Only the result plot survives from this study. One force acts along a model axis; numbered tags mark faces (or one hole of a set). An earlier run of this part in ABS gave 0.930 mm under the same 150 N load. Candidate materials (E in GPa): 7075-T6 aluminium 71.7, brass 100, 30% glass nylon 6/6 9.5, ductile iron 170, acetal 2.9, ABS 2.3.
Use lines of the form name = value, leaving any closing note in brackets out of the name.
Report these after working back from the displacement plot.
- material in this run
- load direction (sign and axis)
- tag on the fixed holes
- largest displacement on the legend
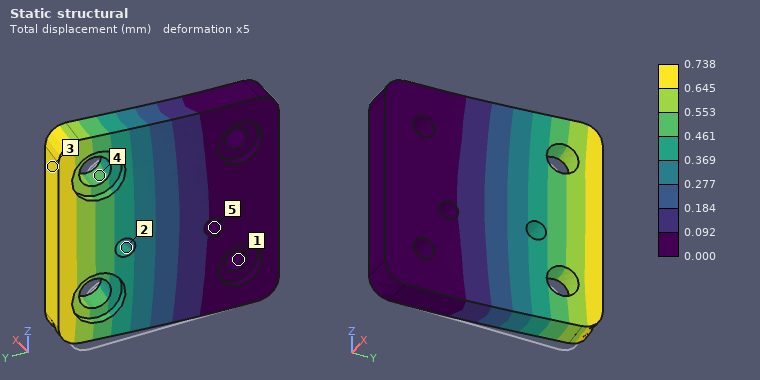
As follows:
material in this run = acetal
load direction = +X
tag on the fixed holes = 1
largest displacement on the legend = 0.738 mm
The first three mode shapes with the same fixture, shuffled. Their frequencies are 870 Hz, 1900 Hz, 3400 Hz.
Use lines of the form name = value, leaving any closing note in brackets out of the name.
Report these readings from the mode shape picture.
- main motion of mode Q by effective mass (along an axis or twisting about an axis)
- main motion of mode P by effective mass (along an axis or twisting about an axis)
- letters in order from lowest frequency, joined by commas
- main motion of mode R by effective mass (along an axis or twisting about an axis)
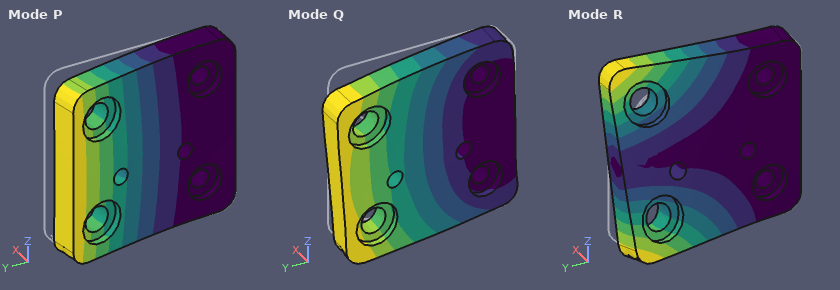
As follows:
main motion of mode Q by effective mass = along Z
main motion of mode P by effective mass = along X
letters in order from lowest frequency, joined by commas = P, R, Q
main motion of mode R by effective mass = twisting about Y
